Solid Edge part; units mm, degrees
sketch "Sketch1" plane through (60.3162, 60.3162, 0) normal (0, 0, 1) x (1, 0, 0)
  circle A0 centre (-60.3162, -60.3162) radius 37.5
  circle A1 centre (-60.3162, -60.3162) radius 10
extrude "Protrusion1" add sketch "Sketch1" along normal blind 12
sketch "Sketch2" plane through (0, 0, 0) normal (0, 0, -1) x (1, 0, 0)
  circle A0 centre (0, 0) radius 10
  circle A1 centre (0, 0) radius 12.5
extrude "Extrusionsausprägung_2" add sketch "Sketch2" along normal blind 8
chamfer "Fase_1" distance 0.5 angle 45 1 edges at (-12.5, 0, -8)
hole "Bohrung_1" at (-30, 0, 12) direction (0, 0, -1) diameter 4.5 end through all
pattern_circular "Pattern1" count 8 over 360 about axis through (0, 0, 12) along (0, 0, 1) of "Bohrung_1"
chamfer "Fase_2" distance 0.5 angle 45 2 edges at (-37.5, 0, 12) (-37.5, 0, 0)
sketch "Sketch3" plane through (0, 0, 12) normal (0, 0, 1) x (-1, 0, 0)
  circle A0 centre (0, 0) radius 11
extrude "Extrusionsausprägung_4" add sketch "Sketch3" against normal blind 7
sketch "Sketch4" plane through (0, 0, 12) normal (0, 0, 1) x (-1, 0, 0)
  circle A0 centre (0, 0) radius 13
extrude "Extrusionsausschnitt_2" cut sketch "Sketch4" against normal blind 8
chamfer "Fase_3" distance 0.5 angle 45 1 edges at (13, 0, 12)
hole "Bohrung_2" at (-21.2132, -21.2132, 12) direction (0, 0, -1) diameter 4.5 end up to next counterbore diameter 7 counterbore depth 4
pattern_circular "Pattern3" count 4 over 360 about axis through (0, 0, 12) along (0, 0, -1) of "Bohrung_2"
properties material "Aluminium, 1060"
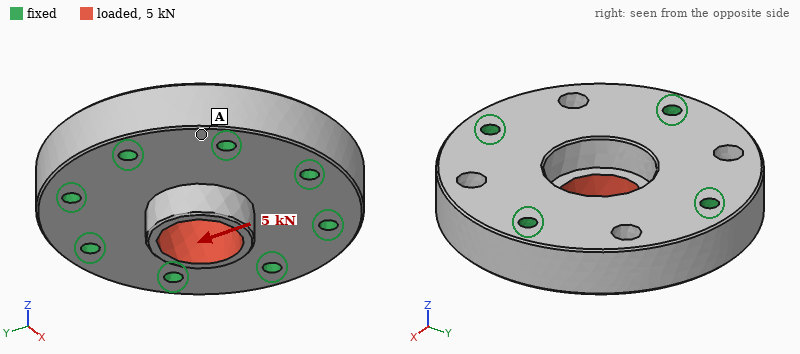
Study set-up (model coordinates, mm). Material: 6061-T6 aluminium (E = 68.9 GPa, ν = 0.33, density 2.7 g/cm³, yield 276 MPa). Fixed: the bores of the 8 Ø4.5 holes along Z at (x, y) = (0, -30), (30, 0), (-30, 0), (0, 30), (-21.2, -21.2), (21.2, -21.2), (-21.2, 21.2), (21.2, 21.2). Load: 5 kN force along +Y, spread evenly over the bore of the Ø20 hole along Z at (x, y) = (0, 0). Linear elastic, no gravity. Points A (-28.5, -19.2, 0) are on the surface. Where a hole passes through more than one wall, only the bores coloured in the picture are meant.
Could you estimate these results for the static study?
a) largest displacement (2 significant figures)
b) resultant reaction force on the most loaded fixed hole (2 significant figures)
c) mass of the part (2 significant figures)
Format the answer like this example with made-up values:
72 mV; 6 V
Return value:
16 µm; 1.1 kN; 130 g
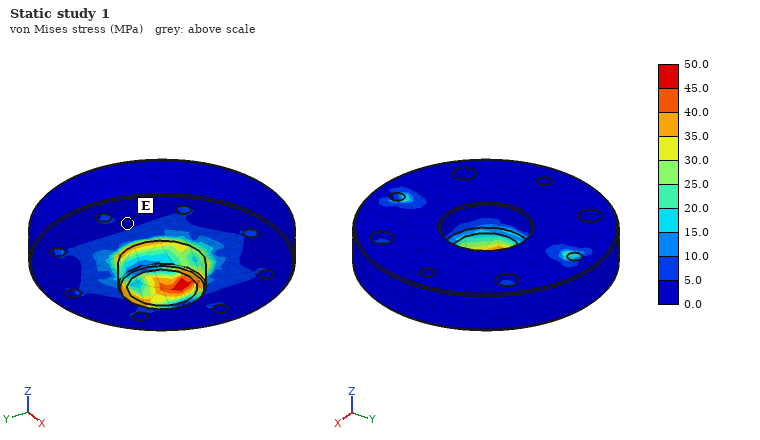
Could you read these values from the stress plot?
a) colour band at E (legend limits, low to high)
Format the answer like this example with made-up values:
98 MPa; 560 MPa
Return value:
0.0 to 5.0 MPa
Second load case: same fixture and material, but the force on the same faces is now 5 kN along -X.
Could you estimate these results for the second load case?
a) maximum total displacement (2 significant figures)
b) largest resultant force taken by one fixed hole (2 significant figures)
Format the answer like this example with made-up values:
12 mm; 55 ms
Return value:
17 µm; 1.2 kN
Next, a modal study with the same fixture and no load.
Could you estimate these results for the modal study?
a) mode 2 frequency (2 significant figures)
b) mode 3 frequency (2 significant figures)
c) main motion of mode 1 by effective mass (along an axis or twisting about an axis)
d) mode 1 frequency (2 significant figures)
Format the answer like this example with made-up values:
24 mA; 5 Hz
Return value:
31 kHz; 31 kHz; along Z; 24 kHz
